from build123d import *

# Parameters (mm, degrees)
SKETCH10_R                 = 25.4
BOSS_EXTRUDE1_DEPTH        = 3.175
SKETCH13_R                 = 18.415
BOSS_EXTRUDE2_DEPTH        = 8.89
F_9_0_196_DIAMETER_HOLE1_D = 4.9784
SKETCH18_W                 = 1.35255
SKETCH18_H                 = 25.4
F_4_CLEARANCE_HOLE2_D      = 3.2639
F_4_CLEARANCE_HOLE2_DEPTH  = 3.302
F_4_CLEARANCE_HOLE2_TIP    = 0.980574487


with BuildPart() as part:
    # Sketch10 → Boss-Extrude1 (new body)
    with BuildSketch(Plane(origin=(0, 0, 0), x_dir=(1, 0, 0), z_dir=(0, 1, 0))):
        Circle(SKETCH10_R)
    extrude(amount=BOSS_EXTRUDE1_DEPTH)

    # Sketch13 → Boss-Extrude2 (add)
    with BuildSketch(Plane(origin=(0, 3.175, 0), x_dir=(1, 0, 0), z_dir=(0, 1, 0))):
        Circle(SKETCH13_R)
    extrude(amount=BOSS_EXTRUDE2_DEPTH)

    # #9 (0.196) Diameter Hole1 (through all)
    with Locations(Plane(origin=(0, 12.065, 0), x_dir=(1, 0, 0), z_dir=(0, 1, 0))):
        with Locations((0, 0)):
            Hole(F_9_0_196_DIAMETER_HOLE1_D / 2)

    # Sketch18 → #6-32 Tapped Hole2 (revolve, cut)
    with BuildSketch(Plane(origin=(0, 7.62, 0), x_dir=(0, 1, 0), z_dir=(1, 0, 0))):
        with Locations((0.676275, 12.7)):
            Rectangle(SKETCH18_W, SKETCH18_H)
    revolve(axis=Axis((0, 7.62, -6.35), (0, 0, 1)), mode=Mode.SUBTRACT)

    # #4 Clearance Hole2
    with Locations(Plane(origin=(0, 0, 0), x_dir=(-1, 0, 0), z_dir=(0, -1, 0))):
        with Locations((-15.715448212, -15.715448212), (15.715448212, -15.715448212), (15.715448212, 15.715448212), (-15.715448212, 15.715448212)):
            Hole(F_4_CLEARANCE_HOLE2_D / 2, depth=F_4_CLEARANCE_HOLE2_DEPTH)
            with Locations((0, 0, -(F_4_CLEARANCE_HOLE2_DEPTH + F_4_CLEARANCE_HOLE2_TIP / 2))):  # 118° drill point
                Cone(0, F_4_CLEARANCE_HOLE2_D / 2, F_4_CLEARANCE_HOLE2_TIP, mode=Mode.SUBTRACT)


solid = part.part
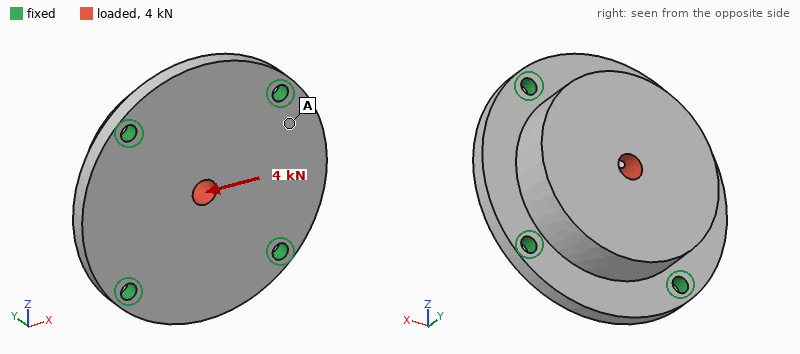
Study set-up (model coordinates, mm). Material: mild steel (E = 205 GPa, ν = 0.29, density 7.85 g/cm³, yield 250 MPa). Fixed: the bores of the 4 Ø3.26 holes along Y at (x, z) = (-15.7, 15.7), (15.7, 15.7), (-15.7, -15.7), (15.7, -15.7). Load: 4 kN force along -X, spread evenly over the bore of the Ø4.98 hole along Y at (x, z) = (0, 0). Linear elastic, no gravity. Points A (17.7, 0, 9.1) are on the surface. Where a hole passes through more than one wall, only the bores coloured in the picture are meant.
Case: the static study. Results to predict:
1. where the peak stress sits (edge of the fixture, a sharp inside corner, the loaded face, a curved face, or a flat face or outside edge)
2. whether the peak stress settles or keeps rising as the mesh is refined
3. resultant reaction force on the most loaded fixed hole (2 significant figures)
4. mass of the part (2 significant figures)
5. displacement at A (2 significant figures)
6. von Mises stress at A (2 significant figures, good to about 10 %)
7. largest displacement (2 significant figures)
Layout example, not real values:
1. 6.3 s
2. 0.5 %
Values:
1. edge of the fixture
2. keeps rising
3. 1.1 kN
4. 120 g
5. 1.5 µm
6. 10 MPa
7. 3.0 µm
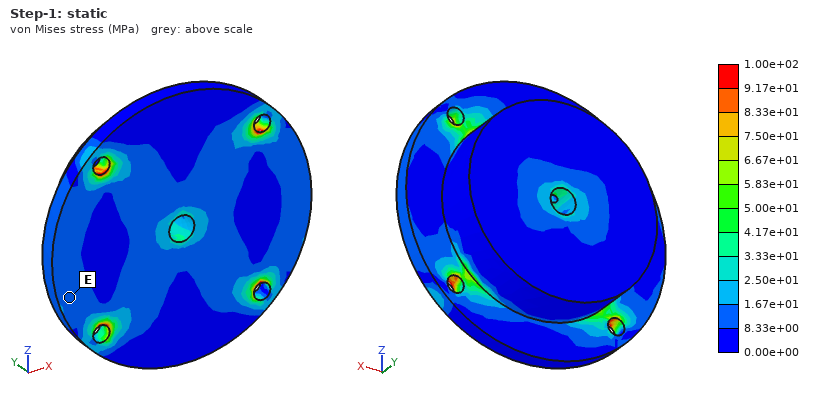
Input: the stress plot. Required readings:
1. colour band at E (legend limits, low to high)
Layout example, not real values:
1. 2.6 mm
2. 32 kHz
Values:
1. 8.33e+00 to 1.67e+01 MPa
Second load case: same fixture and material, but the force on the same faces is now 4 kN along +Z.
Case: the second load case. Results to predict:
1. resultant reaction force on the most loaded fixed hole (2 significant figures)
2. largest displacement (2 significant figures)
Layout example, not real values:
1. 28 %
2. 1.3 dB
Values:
1. 1.1 kN
2. 3.0 µm
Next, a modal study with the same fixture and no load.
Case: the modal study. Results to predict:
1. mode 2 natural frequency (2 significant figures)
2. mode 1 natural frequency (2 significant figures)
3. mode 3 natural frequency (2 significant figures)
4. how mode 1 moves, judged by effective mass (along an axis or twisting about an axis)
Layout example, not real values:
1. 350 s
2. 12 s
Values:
1. 18 kHz
2. 14 kHz
3. 18 kHz
4. along Y
